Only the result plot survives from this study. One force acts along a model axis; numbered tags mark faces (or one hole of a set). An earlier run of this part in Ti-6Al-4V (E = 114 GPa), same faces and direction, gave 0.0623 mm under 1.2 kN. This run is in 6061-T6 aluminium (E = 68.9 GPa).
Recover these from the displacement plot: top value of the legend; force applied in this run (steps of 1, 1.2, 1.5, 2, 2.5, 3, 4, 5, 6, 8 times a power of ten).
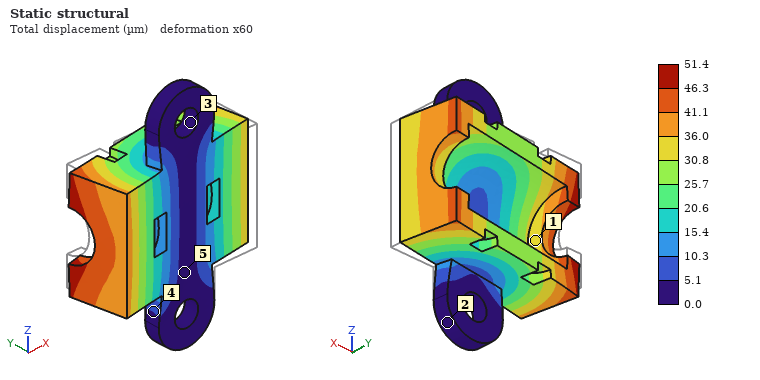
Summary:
51.4 µm
600 N
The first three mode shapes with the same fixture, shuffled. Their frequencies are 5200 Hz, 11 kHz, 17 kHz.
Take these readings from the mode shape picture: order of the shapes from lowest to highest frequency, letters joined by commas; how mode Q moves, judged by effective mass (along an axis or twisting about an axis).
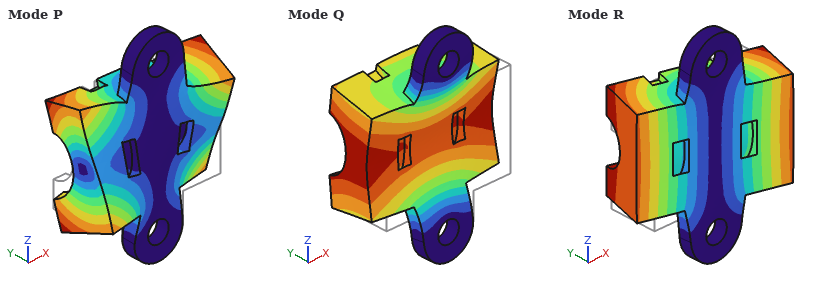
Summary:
R, Q, P
along Y
